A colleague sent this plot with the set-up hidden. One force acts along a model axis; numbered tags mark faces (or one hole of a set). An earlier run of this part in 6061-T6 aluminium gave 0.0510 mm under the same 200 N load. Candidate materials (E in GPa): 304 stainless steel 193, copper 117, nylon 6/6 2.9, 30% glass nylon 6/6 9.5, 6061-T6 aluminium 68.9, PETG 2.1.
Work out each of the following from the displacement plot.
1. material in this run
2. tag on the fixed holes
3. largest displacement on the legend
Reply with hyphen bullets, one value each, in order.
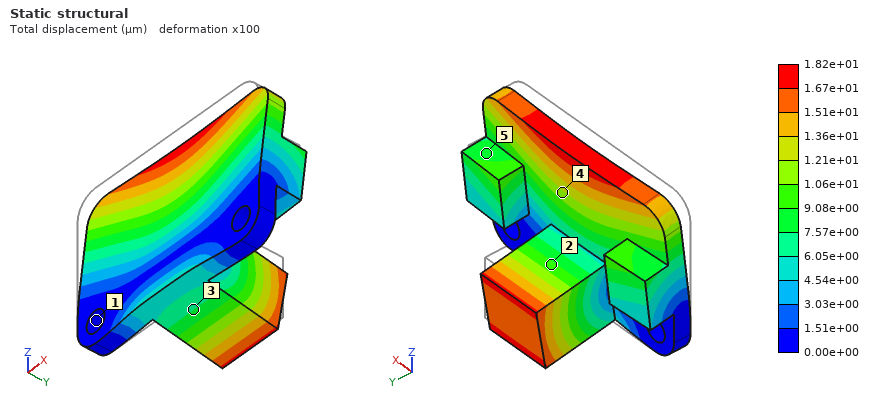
- 304 stainless steel
- 1
- 1.82e+01 µm
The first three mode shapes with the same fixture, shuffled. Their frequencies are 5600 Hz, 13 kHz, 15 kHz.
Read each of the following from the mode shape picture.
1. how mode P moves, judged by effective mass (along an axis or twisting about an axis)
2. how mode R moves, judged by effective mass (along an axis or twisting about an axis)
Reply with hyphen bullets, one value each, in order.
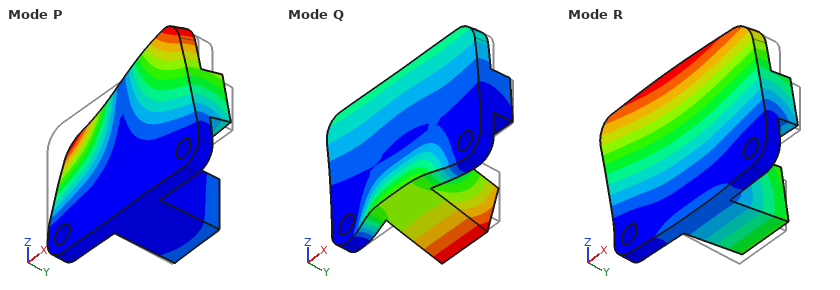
- twisting about Z
- along Y
